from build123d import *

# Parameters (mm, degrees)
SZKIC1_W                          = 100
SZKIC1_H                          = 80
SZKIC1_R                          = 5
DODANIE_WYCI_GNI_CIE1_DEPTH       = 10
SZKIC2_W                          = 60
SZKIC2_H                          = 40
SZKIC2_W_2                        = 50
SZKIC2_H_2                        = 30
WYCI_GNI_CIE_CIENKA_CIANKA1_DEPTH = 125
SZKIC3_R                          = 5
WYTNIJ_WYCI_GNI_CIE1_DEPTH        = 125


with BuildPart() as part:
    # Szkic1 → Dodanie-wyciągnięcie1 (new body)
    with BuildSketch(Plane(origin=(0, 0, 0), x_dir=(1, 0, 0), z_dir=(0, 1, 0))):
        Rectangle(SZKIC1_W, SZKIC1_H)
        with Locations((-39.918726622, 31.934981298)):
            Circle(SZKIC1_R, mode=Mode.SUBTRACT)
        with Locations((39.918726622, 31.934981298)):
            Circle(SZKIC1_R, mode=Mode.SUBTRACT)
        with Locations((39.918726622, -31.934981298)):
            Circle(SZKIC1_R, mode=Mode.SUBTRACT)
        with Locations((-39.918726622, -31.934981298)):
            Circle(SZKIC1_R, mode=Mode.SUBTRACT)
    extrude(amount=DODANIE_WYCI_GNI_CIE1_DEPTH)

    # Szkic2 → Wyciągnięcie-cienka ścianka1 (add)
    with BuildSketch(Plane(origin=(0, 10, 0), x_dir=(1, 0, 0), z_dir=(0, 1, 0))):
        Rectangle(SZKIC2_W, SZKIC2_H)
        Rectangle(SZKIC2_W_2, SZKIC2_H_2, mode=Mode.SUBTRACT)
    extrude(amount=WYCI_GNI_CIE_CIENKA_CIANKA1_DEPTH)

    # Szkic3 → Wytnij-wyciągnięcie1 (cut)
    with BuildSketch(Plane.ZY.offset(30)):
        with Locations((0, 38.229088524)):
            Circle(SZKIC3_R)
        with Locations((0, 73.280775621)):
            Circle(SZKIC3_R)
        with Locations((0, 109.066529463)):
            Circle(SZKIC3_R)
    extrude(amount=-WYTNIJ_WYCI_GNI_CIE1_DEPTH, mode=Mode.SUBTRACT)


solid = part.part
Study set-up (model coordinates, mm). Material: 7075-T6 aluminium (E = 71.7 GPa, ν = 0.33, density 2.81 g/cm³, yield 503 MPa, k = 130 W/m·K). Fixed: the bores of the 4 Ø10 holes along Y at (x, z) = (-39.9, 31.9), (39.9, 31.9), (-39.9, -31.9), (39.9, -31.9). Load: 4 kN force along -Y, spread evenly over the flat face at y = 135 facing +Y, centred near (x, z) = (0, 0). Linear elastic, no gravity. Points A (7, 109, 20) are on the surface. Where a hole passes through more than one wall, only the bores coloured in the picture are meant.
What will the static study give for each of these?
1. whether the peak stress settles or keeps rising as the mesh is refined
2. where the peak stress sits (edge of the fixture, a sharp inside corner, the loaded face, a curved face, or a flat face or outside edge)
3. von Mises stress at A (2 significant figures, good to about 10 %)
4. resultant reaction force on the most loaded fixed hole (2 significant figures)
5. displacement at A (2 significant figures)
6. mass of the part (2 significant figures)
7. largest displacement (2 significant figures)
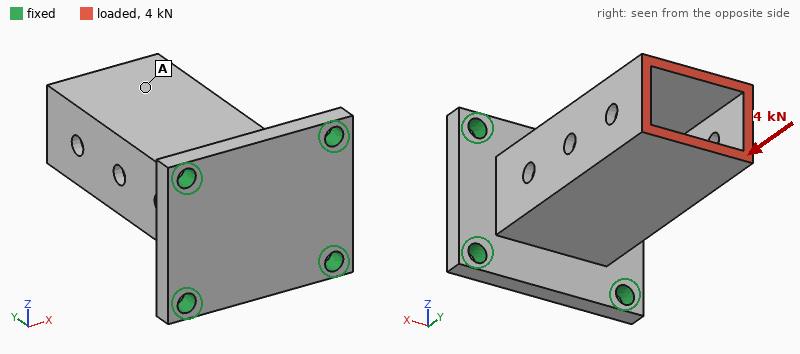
keeps rising
edge of the fixture
4.4 MPa
1.0 kN
15 µm
530 g
17 µm
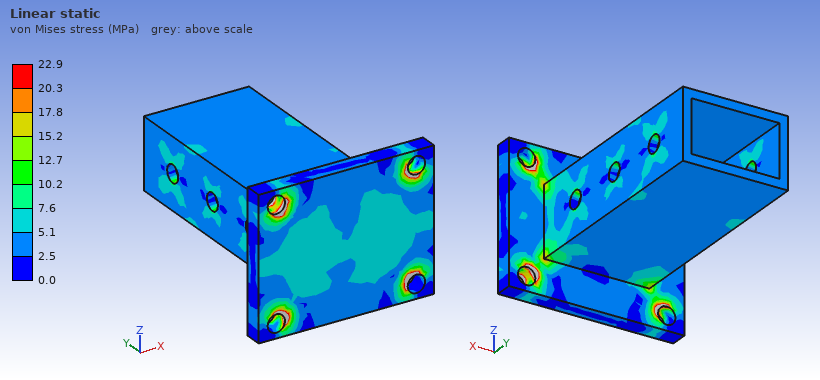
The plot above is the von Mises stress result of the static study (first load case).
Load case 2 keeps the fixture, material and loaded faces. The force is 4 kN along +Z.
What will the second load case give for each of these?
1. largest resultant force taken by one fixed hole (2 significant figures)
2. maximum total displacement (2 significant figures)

5.0 kN
0.54 mm
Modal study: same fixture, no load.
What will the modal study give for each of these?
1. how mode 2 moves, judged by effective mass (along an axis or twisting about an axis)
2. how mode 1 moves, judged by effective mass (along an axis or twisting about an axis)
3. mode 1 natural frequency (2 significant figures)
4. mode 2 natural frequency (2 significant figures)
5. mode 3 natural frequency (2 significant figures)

along X
along Z
1500 Hz
2000 Hz
3600 Hz
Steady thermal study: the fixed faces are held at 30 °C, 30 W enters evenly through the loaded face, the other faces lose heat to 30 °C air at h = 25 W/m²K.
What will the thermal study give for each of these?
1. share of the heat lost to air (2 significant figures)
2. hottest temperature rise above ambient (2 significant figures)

49 %
25 K
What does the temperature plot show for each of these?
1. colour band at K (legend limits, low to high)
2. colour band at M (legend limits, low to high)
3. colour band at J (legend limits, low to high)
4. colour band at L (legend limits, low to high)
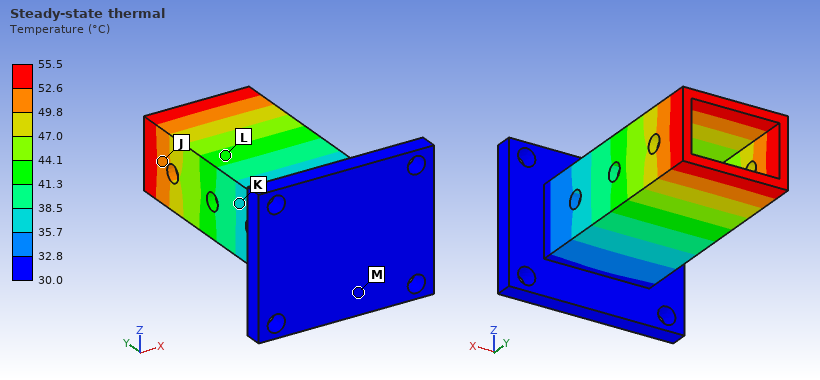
35.7 to 38.5 °C
30.0 to 32.8 °C
49.8 to 52.6 °C
41.3 to 44.1 °C
